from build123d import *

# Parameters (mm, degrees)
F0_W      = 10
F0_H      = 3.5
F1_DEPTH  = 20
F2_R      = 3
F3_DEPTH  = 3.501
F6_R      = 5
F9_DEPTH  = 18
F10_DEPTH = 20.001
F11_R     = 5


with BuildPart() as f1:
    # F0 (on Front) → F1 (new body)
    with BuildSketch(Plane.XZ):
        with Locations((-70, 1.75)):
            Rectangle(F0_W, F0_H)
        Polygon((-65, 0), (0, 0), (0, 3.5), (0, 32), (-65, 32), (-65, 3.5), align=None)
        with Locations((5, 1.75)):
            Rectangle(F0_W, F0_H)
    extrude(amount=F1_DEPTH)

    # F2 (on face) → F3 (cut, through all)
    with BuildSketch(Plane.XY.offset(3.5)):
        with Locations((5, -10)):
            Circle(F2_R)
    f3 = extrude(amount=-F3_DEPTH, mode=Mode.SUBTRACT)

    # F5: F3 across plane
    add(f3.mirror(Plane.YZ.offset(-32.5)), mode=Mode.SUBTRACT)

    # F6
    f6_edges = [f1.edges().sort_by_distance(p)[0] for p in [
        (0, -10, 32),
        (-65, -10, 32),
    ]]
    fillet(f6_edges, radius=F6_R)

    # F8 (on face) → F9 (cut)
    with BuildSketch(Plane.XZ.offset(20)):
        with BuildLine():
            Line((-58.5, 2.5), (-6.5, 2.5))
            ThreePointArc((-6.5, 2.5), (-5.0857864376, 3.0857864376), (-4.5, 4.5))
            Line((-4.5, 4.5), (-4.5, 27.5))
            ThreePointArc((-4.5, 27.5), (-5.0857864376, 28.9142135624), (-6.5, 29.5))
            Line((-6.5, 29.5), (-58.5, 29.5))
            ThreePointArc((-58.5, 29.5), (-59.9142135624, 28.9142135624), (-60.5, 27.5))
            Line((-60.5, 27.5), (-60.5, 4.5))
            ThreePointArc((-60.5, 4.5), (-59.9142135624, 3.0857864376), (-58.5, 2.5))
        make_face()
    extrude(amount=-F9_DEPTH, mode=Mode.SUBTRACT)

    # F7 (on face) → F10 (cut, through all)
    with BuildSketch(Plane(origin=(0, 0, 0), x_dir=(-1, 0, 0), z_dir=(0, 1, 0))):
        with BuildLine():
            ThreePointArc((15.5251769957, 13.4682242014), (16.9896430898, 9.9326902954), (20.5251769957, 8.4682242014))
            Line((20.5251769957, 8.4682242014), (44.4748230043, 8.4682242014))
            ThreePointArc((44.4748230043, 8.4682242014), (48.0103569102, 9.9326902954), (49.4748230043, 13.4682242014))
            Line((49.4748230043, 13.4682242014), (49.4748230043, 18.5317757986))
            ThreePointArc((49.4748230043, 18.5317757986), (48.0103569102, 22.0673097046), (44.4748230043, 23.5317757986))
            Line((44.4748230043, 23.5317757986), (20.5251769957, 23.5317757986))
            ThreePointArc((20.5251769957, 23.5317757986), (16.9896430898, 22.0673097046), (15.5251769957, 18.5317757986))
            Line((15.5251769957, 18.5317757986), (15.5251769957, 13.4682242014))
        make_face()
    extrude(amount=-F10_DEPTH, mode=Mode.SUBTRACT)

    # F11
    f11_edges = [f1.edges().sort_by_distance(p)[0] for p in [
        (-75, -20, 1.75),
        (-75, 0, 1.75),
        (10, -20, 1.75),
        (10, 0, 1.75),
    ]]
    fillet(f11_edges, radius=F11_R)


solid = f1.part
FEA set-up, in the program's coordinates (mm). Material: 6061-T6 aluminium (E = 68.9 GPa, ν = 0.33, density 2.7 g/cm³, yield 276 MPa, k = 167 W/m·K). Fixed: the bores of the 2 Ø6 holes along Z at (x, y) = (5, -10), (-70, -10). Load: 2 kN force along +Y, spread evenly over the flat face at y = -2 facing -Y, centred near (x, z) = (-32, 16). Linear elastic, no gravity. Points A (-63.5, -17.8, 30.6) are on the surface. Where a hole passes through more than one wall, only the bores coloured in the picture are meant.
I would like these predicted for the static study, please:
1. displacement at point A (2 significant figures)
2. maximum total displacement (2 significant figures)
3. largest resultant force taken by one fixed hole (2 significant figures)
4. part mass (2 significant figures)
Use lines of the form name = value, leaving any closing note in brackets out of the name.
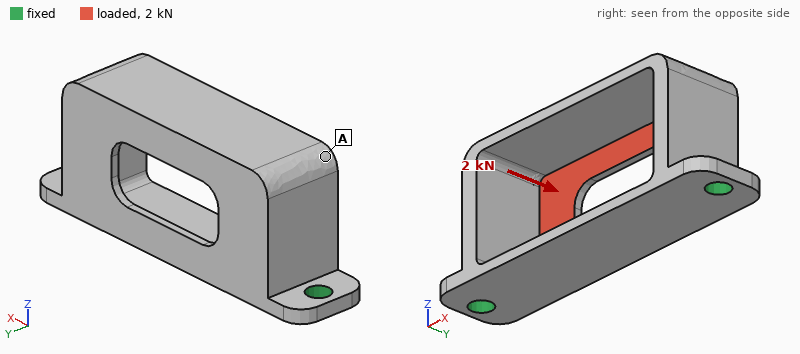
displacement at point A = 0.21 mm
maximum total displacement = 0.23 mm
largest resultant force taken by one fixed hole = 1.0 kN
part mass = 39 g
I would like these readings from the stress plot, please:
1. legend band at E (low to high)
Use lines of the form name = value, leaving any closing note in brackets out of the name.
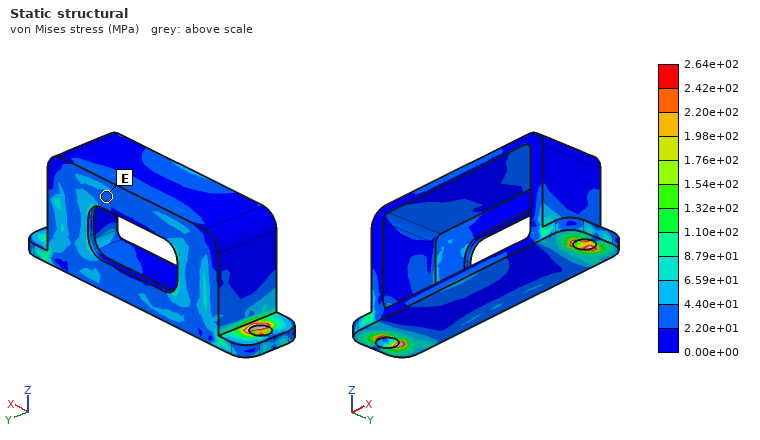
legend band at E = 2.20e+01 to 4.40e+01 MPa
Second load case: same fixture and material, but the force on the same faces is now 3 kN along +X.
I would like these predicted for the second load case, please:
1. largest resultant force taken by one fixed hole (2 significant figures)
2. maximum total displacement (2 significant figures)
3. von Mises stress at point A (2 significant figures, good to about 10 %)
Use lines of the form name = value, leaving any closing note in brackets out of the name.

largest resultant force taken by one fixed hole = 1.6 kN
maximum total displacement = 0.12 mm
von Mises stress at point A = 12 MPa
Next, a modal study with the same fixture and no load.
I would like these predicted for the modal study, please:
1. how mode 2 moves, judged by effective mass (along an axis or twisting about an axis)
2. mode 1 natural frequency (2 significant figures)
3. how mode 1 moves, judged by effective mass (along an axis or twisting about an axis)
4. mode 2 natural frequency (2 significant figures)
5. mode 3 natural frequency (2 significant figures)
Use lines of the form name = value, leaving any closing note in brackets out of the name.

how mode 2 moves, judged by effective mass = along X
mode 1 natural frequency = 2800 Hz
how mode 1 moves, judged by effective mass = along Y
mode 2 natural frequency = 3600 Hz
mode 3 natural frequency = 5400 Hz
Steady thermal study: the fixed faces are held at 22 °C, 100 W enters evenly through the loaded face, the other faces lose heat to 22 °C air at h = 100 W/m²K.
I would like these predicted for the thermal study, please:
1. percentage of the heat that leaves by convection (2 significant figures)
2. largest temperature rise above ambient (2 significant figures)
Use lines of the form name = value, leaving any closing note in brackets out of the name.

percentage of the heat that leaves by convection = 34 %
largest temperature rise above ambient = 63 K
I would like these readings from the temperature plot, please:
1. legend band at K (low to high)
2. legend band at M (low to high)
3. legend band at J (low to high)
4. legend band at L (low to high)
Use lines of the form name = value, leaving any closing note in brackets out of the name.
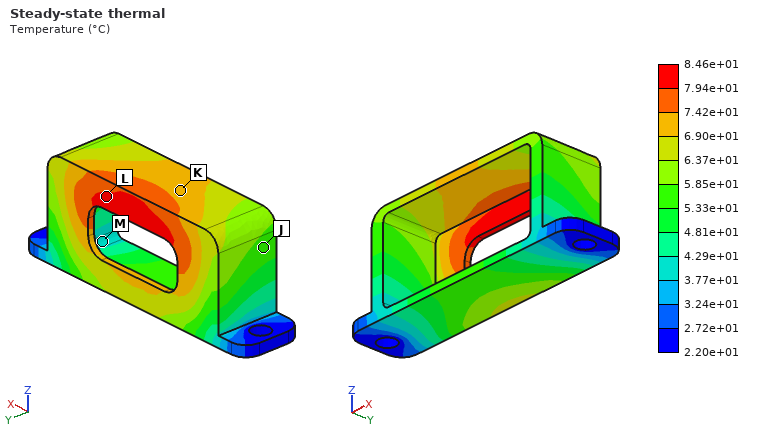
legend band at K = 6.90e+01 to 7.42e+01 °C
legend band at M = 3.77e+01 to 4.29e+01 °C
legend band at J = 5.33e+01 to 5.85e+01 °C
legend band at L = 7.94e+01 to 8.46e+01 °C
